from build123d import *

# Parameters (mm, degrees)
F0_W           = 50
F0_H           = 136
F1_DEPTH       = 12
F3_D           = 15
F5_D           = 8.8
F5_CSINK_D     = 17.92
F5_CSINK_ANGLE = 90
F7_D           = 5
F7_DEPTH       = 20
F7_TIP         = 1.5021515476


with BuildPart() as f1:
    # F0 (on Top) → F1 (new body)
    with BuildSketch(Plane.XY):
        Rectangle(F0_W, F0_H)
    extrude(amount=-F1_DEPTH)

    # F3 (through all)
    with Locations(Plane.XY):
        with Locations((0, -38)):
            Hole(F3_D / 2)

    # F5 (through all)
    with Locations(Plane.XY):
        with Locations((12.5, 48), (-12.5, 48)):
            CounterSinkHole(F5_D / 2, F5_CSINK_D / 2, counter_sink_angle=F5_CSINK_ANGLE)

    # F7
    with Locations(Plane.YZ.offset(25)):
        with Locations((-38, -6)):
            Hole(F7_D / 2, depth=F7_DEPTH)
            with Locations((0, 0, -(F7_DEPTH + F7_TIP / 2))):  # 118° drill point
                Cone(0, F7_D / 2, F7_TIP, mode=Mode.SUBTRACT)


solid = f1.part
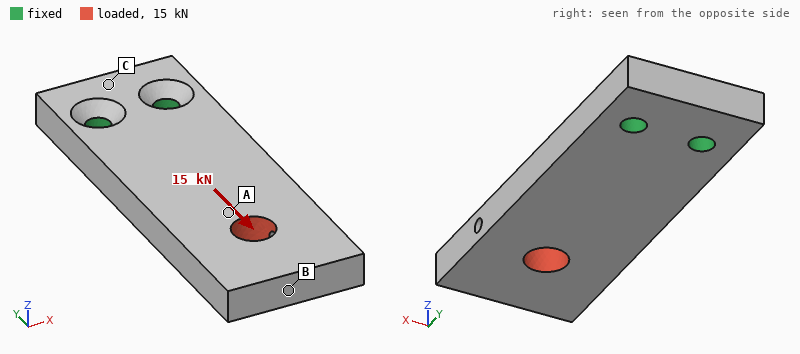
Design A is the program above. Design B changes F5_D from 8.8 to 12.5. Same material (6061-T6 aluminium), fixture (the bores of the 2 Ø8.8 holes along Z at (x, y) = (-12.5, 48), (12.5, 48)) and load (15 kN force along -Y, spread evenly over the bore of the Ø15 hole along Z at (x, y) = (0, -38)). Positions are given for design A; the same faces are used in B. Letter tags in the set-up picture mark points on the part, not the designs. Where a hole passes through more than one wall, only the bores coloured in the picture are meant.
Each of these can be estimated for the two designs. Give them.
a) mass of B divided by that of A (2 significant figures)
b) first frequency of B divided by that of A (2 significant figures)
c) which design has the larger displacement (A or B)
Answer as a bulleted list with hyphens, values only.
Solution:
- 0.99
- 1.1
- A
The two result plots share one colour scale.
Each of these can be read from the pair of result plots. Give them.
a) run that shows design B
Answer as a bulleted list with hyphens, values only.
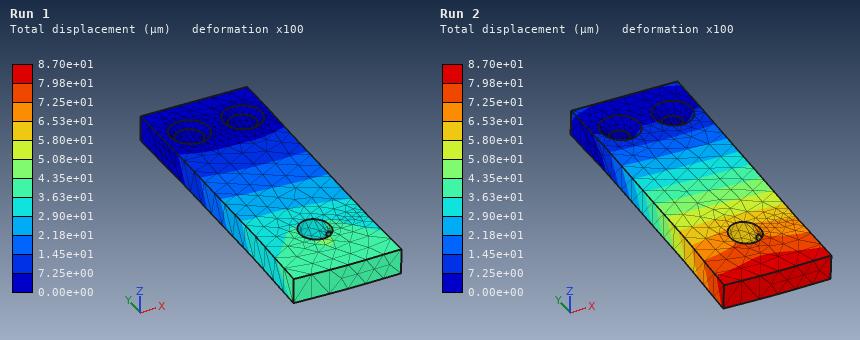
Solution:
- Run 1
